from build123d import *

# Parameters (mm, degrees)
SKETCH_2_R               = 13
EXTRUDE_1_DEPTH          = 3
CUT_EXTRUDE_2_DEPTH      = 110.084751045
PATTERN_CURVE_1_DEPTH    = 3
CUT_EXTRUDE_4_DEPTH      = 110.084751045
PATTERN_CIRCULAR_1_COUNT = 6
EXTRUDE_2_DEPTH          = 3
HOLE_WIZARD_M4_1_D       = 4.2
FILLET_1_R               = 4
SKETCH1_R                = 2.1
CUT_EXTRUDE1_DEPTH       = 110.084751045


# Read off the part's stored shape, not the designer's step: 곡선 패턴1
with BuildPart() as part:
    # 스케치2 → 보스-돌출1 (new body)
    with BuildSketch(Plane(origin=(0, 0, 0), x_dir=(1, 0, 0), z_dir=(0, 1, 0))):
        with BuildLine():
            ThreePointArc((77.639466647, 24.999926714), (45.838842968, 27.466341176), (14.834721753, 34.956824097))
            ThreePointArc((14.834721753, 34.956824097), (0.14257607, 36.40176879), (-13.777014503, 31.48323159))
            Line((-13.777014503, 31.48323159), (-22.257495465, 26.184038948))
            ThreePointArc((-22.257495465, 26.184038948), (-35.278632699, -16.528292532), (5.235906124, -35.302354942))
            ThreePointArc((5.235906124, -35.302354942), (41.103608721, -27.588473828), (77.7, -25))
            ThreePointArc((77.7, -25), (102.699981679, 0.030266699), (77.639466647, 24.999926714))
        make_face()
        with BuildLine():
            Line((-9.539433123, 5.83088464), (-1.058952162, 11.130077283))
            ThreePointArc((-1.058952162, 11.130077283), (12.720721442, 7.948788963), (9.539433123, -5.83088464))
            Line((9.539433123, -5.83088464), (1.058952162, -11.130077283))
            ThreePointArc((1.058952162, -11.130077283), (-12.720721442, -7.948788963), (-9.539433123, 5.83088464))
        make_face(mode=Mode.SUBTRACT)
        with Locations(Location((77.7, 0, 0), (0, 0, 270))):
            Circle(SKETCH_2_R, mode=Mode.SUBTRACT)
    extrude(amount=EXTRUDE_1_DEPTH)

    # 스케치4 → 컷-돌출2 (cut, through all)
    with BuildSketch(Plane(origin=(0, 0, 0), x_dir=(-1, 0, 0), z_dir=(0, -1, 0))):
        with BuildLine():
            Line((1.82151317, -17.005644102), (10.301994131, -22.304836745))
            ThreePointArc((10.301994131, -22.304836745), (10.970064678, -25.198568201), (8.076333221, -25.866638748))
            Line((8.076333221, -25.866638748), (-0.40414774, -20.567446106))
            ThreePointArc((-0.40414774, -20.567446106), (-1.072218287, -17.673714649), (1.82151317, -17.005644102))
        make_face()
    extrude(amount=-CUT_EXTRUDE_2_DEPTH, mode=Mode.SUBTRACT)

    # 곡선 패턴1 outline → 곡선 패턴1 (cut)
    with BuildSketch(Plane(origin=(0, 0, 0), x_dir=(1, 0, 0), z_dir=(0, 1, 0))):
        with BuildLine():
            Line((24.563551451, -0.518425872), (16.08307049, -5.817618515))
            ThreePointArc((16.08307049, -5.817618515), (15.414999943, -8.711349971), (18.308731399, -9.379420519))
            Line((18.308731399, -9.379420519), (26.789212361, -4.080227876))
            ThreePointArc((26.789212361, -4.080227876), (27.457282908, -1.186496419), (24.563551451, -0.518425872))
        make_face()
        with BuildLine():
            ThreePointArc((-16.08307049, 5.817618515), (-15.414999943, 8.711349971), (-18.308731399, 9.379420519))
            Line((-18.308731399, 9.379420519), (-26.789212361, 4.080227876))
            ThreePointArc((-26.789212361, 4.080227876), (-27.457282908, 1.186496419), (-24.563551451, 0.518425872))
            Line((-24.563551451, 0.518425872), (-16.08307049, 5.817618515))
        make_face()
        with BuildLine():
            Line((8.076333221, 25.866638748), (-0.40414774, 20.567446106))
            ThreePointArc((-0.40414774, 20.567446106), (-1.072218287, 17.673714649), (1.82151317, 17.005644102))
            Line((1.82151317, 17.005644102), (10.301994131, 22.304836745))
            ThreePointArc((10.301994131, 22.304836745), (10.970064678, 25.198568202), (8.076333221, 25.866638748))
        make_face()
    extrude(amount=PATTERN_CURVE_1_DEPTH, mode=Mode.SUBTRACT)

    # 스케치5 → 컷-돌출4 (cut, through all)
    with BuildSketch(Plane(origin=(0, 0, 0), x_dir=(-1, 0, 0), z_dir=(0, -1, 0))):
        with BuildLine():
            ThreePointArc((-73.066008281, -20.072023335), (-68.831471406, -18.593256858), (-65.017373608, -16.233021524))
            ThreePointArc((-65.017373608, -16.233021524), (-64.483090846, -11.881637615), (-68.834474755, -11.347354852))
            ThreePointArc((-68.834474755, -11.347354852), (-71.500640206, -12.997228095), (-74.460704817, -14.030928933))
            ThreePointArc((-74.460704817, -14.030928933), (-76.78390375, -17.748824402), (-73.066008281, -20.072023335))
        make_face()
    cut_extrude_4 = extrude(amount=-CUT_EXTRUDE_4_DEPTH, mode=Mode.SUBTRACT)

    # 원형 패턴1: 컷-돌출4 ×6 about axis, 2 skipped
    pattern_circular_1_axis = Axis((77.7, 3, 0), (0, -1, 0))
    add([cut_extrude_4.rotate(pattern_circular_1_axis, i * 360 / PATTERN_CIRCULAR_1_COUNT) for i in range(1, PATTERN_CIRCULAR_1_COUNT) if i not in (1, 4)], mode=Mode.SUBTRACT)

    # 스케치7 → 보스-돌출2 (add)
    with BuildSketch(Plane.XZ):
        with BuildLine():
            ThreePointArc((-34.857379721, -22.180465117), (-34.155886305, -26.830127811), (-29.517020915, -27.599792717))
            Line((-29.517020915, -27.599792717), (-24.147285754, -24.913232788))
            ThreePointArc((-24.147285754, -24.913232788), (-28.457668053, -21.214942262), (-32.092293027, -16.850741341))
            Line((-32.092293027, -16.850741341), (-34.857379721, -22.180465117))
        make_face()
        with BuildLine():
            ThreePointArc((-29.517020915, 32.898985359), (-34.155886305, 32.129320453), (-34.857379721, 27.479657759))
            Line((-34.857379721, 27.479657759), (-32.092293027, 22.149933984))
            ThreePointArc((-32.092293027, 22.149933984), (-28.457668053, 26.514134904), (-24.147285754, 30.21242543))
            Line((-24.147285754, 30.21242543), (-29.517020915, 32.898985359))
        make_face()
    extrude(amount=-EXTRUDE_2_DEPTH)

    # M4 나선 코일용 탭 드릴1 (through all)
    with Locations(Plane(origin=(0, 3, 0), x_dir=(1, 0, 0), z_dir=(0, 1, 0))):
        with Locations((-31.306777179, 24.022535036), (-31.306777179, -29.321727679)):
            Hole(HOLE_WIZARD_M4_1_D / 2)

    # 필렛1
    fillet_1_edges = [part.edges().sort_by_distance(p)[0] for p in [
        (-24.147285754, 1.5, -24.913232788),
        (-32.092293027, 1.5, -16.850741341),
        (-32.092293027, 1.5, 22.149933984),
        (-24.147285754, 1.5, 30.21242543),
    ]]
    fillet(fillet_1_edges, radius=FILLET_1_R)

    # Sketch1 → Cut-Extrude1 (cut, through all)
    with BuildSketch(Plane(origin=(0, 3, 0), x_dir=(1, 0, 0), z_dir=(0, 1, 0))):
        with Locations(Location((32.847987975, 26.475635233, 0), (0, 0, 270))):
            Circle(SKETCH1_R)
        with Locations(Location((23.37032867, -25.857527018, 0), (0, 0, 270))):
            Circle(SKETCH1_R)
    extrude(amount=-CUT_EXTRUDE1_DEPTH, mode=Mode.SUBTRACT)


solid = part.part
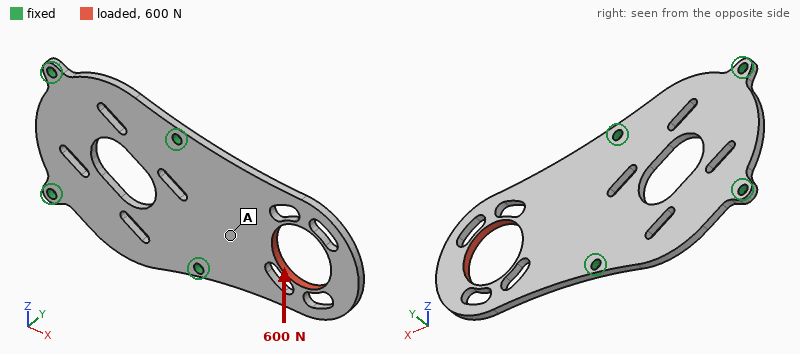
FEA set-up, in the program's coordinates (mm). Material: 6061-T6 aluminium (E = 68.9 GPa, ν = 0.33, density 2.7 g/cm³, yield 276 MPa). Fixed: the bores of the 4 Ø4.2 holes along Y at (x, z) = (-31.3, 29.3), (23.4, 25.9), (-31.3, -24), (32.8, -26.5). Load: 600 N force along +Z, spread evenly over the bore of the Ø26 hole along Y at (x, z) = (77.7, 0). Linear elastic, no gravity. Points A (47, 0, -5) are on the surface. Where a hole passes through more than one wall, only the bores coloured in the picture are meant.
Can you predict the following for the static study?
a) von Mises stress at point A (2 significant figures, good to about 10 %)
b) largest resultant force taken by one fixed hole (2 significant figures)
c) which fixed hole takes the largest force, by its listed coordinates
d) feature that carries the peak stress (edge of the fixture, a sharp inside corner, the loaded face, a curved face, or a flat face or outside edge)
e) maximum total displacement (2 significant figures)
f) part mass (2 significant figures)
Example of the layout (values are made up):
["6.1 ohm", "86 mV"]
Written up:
["9.8 MPa", "670 N", "(32.8, -26.5)", "a curved face", "58 µm", "50 g"]
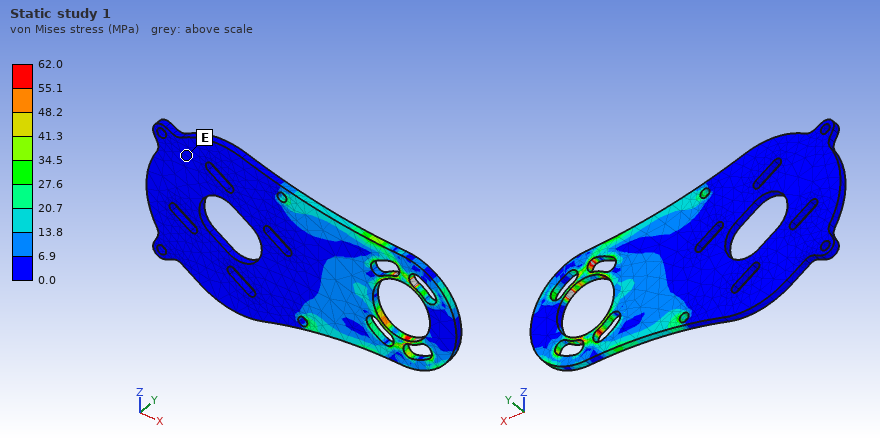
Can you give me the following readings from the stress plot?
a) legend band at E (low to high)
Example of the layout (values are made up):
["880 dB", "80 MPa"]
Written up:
["0.0 to 6.9 MPa"]
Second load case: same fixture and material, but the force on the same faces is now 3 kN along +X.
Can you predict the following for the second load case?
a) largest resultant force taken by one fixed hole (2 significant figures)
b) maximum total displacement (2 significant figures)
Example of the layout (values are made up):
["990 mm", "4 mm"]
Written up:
["1.4 kN", "84 µm"]
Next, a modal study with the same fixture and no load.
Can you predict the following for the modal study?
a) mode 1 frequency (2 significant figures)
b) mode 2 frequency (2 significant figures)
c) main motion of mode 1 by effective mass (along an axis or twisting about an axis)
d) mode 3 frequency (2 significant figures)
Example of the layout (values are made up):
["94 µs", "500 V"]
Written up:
["570 Hz", "1800 Hz", "along Y", "2300 Hz"]
